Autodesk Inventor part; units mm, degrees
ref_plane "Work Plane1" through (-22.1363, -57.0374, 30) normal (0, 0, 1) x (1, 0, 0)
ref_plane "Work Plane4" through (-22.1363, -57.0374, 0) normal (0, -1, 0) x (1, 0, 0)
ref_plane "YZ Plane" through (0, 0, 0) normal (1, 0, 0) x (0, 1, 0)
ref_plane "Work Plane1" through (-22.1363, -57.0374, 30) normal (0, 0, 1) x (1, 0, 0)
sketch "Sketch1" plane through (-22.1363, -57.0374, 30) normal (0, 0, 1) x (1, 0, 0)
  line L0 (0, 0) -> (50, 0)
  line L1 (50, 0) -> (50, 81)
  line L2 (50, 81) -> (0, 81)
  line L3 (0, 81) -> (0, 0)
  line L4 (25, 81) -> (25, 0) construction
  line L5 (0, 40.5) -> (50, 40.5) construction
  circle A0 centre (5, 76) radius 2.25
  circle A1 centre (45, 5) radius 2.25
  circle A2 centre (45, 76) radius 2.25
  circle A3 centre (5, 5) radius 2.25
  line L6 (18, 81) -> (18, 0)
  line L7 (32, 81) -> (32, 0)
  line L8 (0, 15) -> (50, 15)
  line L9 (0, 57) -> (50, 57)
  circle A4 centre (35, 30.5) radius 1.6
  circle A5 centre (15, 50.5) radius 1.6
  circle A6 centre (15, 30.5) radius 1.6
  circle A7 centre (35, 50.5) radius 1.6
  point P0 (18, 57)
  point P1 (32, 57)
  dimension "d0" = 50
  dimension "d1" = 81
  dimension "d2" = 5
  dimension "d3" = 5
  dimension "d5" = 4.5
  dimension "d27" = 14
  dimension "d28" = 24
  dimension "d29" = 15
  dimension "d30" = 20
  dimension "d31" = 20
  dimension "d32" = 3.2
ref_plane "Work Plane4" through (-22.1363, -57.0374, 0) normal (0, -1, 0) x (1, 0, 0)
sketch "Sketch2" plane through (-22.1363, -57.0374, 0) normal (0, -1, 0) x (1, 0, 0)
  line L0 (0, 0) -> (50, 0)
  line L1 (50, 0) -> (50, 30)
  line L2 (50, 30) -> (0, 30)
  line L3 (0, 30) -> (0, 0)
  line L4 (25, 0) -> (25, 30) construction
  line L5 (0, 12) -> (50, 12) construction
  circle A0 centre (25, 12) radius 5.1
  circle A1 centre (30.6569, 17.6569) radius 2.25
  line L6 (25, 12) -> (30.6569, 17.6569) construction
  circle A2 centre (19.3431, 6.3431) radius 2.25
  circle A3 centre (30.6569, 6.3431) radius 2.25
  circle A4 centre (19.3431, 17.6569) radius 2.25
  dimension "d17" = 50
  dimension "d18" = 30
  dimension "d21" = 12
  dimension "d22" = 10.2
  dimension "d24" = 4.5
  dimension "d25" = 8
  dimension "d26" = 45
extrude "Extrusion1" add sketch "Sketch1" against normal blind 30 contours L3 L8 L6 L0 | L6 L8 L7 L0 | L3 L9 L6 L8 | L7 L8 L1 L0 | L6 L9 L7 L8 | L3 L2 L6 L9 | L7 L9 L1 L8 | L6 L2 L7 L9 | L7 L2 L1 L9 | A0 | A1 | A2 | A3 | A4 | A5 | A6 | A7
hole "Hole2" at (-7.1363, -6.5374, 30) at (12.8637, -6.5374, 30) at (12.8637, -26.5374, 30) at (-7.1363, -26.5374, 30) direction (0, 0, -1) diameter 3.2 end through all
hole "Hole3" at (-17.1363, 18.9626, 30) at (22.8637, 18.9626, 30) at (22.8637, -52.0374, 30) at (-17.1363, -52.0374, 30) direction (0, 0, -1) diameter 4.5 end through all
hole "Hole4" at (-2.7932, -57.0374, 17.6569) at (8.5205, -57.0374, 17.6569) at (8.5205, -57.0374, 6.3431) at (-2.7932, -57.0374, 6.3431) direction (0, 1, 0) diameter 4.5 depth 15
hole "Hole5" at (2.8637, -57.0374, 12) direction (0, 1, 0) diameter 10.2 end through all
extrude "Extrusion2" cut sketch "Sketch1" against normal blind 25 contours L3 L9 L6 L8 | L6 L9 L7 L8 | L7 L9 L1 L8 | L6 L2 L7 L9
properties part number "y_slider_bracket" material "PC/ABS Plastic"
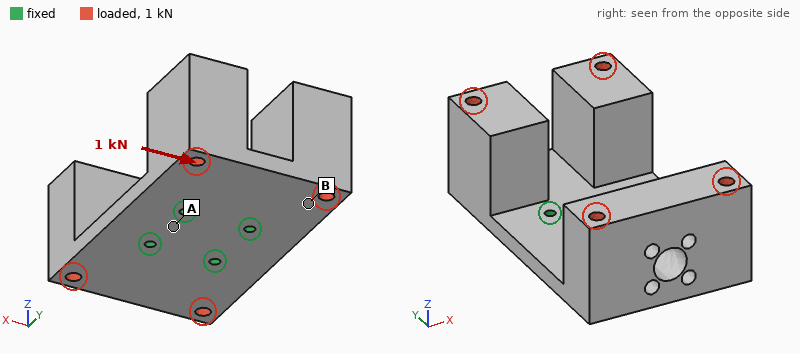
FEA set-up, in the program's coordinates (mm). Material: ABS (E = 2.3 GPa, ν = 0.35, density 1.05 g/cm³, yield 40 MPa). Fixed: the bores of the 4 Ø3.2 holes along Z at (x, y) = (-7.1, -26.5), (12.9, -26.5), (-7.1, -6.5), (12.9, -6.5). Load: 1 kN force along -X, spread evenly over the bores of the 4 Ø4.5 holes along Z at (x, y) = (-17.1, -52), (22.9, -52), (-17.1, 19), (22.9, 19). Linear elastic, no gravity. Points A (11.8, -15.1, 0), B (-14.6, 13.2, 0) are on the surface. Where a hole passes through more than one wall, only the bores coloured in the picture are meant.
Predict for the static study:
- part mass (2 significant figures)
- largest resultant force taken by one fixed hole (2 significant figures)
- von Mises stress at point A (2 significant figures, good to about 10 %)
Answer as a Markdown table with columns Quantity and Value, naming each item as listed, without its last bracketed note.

| Quantity | Value |
|---|---|
| part mass | 59 g |
| largest resultant force taken by one fixed hole | 370 N |
| von Mises stress at point A | 5.1 MPa |
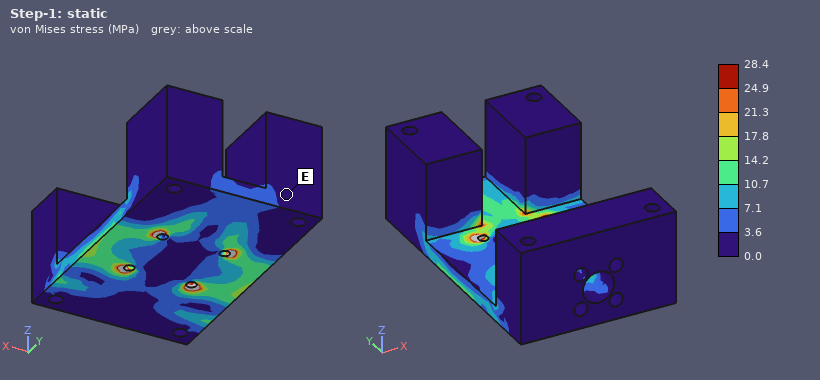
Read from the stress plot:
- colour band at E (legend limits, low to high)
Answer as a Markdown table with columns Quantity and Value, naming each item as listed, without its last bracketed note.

| Quantity | Value |
|---|---|
| colour band at E | 0.0 to 3.6 MPa |
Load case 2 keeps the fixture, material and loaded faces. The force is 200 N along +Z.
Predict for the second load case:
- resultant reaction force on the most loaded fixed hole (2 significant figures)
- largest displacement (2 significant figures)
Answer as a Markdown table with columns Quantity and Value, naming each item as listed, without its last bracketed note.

| Quantity | Value |
|---|---|
| resultant reaction force on the most loaded fixed hole | 51 N |
| largest displacement | 0.99 mm |
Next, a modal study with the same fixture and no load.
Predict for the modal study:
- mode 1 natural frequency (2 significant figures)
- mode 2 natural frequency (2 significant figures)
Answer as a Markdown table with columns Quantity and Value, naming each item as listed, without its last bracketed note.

| Quantity | Value |
|---|---|
| mode 1 natural frequency | 400 Hz |
| mode 2 natural frequency | 470 Hz |
